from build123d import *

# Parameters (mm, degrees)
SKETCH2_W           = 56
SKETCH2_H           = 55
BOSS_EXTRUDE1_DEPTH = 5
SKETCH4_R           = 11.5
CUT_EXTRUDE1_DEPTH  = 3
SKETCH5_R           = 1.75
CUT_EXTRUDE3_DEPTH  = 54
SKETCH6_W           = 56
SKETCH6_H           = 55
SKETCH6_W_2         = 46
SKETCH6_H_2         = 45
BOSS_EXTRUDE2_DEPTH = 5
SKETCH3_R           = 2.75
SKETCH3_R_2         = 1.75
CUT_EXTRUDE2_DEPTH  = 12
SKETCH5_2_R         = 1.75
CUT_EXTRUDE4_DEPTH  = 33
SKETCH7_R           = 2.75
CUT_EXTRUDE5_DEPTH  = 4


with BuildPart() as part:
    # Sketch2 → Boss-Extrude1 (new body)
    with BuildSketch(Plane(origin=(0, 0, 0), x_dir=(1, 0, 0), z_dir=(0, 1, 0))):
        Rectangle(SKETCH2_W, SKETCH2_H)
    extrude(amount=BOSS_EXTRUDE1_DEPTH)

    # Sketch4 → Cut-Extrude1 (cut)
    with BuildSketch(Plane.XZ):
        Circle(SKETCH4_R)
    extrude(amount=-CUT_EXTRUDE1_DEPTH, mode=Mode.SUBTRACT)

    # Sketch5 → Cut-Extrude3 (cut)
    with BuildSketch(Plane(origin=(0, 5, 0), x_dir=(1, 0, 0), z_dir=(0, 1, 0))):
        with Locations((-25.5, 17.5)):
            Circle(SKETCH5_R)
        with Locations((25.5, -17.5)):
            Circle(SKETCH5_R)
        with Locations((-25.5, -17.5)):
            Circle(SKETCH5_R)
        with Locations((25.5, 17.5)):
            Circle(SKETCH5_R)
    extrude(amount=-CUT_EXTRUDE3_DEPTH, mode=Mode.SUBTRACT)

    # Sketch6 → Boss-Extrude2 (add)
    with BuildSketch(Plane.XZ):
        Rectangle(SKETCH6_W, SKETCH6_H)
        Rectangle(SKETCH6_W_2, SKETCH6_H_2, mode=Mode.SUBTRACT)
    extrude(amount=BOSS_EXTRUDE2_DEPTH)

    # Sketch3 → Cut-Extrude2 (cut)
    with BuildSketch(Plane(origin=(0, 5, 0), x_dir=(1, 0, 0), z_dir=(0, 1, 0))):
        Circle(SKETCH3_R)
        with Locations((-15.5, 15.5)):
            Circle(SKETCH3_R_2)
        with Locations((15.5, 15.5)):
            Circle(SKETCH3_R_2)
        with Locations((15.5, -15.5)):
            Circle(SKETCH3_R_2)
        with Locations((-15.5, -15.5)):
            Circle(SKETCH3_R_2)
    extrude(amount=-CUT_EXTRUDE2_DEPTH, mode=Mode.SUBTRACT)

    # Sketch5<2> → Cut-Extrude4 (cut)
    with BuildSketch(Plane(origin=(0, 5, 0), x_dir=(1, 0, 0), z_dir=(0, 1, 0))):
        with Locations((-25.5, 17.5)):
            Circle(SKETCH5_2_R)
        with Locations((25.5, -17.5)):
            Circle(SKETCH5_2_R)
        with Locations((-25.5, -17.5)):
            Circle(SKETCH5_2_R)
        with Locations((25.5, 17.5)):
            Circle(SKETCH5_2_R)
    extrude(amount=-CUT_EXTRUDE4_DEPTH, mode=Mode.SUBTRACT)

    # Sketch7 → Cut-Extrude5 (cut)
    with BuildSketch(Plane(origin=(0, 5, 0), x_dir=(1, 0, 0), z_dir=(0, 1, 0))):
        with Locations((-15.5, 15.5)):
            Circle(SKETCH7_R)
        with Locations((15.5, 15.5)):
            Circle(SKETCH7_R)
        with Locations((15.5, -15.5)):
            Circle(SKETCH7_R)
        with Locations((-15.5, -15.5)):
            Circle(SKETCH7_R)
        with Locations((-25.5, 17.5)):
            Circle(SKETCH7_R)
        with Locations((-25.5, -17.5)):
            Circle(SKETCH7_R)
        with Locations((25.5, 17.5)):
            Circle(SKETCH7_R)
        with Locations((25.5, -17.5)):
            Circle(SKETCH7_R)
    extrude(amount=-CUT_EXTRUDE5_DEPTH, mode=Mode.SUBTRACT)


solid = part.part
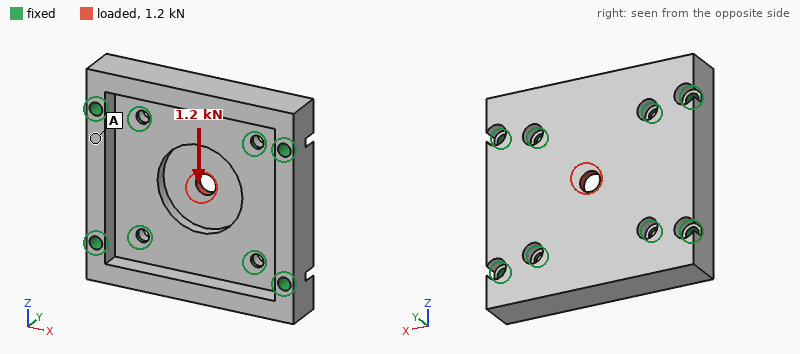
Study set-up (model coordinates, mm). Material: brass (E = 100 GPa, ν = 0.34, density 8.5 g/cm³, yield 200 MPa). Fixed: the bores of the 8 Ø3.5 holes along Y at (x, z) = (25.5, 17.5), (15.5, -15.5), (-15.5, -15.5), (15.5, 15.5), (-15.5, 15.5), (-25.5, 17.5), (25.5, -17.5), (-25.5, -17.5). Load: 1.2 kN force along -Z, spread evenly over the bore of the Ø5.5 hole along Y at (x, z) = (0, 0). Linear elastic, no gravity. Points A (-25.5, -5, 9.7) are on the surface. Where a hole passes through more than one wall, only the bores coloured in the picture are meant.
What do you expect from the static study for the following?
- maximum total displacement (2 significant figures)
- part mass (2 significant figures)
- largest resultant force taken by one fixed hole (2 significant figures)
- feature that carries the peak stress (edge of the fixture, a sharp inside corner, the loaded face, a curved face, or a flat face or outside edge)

4.1 µm
150 g
200 N
the loaded face
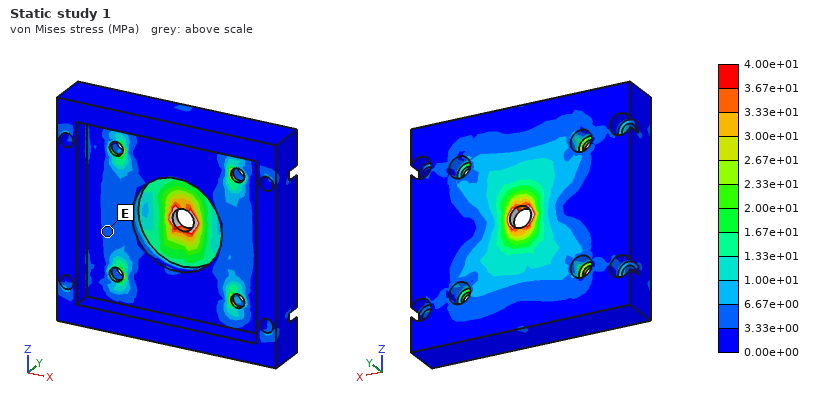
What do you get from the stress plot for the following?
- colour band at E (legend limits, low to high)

3.33e+00 to 6.67e+00 MPa
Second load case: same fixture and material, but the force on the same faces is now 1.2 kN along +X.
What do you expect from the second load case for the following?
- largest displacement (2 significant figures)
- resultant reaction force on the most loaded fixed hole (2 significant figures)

4.0 µm
180 N
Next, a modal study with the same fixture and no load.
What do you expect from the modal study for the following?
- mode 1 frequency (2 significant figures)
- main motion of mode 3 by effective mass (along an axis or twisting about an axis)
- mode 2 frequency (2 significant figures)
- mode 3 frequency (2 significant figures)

9100 Hz
along Y
9100 Hz
11 kHz
